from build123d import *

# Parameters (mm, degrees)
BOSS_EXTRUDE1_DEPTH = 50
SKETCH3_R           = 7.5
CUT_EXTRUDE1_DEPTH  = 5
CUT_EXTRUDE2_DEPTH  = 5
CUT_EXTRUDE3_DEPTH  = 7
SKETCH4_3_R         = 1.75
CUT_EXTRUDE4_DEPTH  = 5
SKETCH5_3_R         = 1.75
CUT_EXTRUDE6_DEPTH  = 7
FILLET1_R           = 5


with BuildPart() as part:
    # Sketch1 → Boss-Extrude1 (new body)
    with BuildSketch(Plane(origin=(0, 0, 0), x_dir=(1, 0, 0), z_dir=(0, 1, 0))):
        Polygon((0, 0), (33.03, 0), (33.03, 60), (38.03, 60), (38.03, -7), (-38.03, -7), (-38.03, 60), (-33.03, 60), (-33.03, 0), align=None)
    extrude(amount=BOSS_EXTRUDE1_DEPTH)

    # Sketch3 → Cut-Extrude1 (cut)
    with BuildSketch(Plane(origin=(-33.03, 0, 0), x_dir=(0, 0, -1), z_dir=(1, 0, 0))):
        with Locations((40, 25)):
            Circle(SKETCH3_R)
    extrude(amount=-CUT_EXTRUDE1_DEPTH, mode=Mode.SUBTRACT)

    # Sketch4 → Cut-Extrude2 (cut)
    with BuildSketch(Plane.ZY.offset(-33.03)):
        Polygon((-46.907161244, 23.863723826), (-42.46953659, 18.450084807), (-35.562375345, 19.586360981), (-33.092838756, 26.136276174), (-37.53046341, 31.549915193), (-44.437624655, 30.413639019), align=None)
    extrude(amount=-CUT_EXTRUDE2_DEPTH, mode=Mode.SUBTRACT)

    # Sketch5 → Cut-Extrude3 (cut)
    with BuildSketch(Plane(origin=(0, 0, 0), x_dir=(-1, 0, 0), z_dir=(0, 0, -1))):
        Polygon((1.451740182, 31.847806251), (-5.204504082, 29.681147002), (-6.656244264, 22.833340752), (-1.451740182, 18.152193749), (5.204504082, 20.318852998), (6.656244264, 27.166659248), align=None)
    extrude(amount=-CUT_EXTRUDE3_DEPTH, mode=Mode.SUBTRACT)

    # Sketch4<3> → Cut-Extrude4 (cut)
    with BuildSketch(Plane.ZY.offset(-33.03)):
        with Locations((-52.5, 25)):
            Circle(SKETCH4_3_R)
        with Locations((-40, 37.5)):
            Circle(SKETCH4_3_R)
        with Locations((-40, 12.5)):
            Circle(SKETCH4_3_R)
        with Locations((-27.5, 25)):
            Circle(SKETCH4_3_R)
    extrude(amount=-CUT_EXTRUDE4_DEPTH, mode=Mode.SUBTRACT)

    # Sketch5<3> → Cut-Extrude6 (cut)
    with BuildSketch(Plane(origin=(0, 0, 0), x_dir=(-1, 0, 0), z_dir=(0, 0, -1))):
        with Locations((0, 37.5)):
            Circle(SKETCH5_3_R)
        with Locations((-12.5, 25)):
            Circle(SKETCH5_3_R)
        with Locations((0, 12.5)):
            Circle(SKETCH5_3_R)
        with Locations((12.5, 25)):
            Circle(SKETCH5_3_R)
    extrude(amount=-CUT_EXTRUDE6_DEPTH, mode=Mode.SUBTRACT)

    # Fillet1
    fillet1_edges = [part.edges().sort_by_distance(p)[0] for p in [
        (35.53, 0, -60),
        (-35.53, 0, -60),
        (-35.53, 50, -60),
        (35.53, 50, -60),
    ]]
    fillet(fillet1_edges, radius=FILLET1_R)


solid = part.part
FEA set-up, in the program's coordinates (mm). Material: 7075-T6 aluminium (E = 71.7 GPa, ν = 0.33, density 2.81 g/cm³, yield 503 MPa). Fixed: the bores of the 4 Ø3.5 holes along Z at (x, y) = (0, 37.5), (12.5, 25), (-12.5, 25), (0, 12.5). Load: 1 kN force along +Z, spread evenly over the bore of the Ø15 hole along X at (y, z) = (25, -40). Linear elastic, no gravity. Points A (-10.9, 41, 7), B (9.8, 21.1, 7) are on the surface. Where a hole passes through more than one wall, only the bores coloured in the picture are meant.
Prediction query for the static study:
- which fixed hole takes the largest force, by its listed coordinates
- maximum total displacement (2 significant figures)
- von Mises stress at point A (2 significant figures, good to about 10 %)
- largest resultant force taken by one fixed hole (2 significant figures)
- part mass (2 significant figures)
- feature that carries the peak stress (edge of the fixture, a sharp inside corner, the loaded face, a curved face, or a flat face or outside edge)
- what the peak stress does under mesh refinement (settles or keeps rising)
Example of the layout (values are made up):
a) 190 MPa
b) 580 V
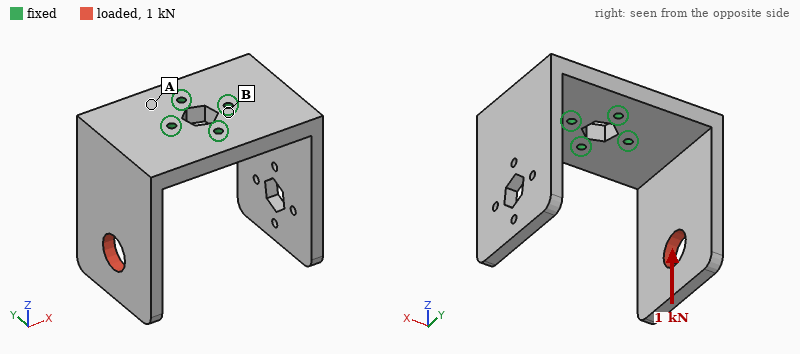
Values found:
a) (-12.5, 25)
b) 0.23 mm
c) 29 MPa
d) 1.5 kN
e) 150 g
f) edge of the fixture
g) keeps rising
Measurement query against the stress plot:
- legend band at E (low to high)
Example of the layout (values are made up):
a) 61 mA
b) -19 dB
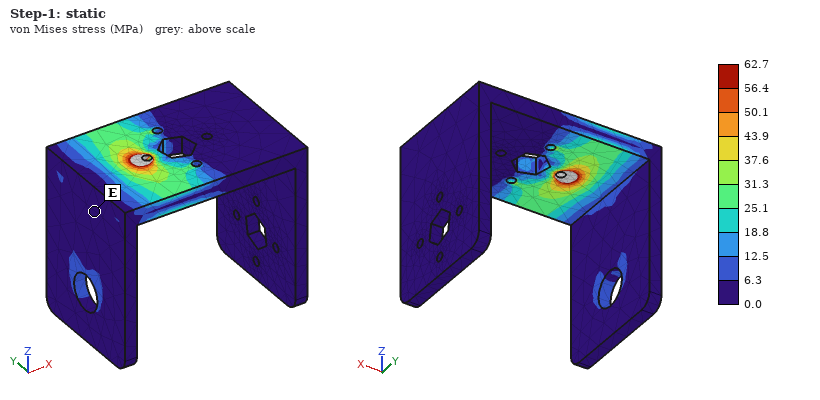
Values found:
a) 0.0 to 6.3 MPa
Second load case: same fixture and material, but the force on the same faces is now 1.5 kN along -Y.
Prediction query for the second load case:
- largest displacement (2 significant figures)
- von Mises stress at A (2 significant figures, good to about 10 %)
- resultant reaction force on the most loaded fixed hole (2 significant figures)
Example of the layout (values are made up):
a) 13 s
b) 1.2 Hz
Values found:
a) 0.71 mm
b) 93 MPa
c) 1.7 kN
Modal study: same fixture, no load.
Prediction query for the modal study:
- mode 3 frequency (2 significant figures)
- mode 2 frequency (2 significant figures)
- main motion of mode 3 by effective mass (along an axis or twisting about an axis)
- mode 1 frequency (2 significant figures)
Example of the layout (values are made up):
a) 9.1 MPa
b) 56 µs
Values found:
a) 1500 Hz
b) 880 Hz
c) twisting about Z
d) 870 Hz
